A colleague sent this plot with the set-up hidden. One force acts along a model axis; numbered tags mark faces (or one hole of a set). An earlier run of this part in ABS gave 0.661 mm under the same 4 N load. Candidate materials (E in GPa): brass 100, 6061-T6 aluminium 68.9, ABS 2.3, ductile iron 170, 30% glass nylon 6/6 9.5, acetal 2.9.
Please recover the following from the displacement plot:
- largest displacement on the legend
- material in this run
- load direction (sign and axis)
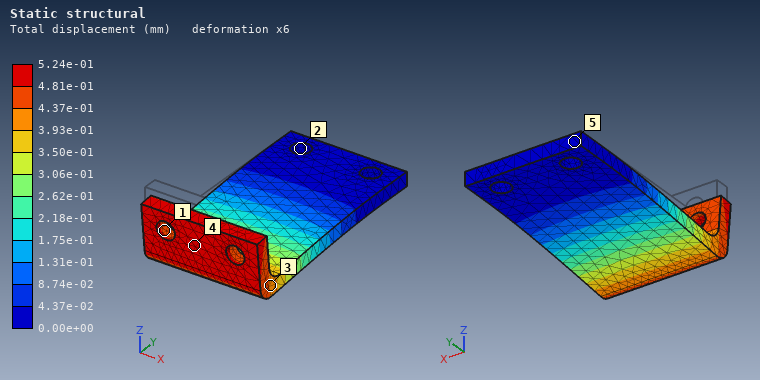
5.24e-01 mm
acetal
-Z
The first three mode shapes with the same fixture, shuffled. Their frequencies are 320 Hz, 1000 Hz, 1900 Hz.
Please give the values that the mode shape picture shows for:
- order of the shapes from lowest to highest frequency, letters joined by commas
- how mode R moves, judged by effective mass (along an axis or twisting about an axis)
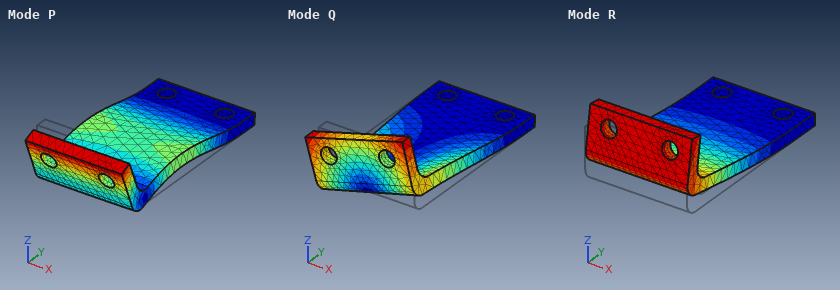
R, Q, P
along Z
